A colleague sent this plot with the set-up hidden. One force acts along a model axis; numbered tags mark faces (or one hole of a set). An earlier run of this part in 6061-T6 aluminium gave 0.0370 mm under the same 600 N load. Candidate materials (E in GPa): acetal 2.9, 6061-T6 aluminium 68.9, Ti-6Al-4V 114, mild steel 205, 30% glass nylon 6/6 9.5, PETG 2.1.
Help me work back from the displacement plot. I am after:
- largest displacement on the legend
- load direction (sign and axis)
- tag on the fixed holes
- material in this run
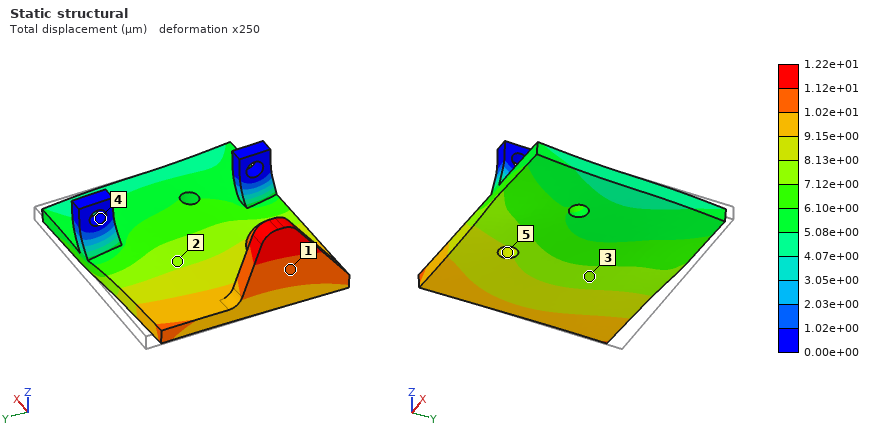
1.22e+01 µm
-Y
4
mild steel
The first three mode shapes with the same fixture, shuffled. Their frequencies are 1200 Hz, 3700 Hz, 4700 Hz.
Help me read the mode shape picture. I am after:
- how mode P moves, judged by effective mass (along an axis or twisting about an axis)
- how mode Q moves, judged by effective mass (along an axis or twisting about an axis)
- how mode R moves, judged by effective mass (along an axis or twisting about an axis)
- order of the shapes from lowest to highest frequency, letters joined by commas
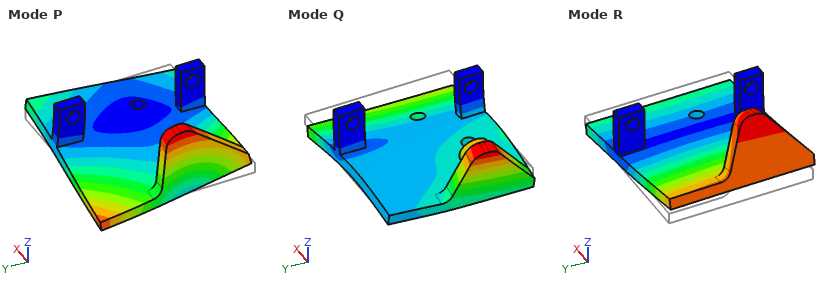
along Y
along X
along Z
R, P, Q
